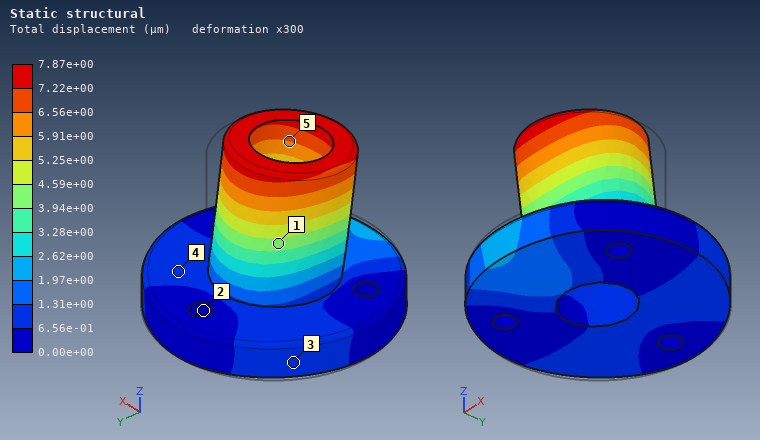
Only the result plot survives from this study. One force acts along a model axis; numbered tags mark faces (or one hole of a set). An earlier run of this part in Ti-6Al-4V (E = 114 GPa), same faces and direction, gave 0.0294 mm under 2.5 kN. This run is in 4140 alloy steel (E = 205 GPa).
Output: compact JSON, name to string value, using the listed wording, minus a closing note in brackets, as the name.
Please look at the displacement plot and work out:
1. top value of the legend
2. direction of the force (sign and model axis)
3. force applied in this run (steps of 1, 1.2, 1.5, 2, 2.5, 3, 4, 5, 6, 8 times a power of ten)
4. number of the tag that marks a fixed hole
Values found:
{"top value of the legend": "7.87e+00 µm", "direction of the force": "-Y", "force applied in this run": "1.2 kN", "number of the tag that marks a fixed hole": "2"}
